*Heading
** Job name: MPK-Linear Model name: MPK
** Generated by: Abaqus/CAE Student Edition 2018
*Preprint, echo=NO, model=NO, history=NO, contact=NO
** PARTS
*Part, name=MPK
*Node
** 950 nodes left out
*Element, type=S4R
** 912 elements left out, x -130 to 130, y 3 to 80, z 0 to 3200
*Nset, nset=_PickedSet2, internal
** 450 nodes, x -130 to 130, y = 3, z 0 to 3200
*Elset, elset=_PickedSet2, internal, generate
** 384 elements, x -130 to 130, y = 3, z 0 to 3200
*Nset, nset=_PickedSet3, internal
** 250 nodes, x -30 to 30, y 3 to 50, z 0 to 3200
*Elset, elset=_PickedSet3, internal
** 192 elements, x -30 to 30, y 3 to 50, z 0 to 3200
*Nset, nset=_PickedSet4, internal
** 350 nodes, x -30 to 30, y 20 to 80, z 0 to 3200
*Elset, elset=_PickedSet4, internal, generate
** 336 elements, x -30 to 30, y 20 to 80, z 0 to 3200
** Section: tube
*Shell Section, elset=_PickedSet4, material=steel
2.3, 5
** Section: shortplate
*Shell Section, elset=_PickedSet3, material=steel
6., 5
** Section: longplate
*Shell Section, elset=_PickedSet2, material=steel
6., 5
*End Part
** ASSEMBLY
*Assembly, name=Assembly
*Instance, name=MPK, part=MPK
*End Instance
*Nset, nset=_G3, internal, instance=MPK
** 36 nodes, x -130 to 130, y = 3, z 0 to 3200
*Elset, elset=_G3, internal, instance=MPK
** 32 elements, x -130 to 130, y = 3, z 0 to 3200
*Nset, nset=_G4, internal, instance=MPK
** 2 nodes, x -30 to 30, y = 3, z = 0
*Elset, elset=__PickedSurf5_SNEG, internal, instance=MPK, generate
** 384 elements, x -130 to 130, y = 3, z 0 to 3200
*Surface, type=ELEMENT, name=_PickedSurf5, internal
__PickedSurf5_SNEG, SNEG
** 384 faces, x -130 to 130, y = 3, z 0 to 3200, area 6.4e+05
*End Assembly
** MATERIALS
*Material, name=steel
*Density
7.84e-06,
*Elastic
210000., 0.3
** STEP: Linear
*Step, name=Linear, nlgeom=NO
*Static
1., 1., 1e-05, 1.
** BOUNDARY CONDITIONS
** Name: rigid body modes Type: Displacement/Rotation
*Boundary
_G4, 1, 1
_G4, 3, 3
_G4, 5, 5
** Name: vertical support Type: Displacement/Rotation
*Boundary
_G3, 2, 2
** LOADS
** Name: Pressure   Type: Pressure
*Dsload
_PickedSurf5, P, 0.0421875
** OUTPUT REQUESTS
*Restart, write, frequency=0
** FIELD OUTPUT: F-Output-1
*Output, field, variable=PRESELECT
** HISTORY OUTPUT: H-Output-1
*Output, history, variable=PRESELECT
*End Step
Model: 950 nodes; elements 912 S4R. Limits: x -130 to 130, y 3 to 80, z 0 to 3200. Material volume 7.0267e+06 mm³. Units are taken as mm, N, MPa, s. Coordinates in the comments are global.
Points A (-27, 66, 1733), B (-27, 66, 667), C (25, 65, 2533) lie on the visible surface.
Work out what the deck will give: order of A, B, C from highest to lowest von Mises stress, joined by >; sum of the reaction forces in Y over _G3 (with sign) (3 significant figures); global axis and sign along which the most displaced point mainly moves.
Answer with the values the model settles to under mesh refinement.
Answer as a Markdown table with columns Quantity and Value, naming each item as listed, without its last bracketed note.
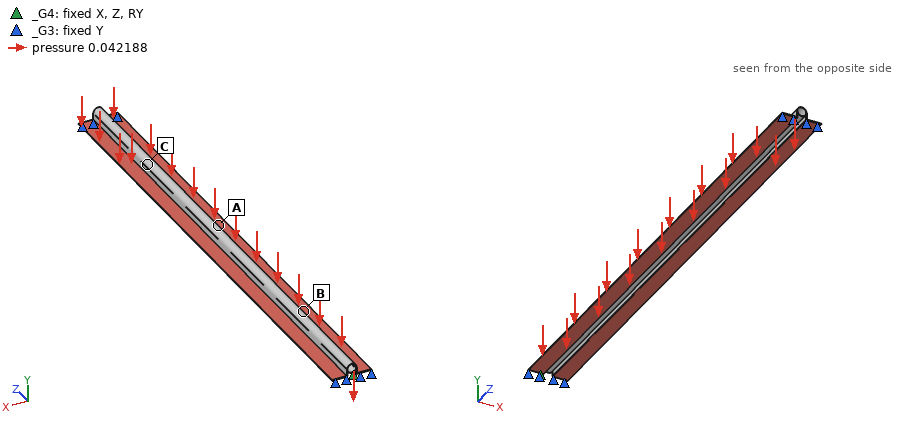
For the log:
| Quantity | Value |
|---|---|
| order of A, B, C from highest to lowest von Mises stress, joined by > | A > B > C |
| sum of the reaction forces in Y over _G3 (with sign) | 27000 N |
| global axis and sign along which the most displaced point mainly moves | -Y |
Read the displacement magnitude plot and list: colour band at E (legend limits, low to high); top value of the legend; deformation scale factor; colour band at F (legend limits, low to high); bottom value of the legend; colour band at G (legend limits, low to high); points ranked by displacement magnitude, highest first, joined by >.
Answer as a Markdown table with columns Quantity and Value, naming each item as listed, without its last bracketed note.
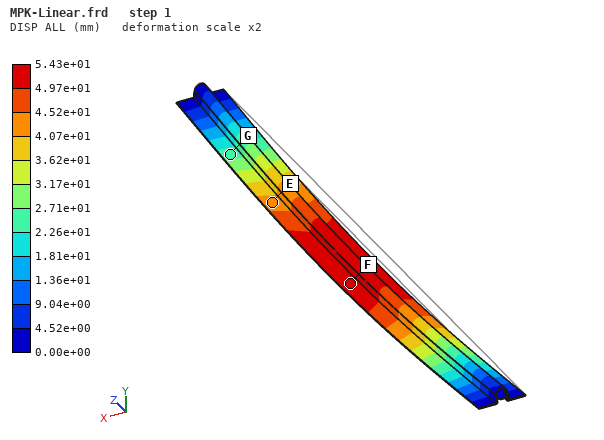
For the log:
| Quantity | Value |
|---|---|
| colour band at E | 4.07e+01 to 4.52e+01 mm |
| top value of the legend | 5.43e+01 mm |
| deformation scale factor | 2 |
| colour band at F | 4.97e+01 to 5.43e+01 mm |
| bottom value of the legend | 0.00e+00 mm |
| colour band at G | 2.26e+01 to 2.71e+01 mm |
| points ranked by displacement magnitude, highest first, joined by > | F > E > G |
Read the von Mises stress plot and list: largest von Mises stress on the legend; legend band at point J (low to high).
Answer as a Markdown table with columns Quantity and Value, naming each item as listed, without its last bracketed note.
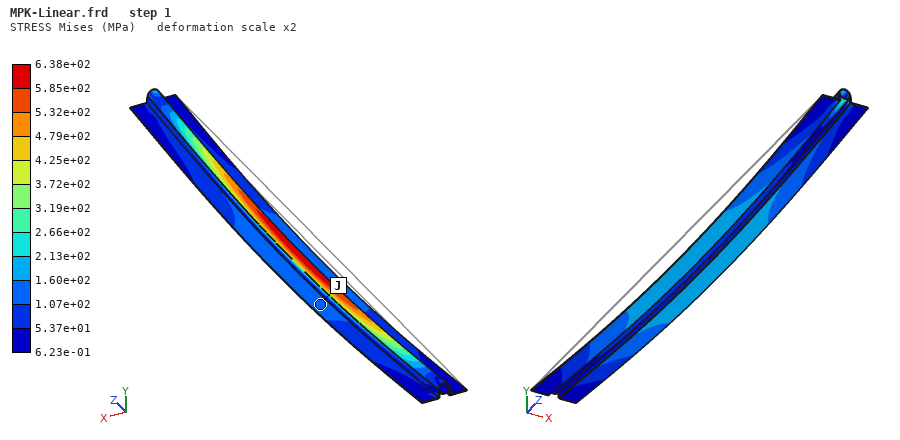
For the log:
| Quantity | Value |
|---|---|
| largest von Mises stress on the legend | 6.38e+02 MPa |
| legend band at point J | 1.07e+02 to 1.60e+02 MPa |
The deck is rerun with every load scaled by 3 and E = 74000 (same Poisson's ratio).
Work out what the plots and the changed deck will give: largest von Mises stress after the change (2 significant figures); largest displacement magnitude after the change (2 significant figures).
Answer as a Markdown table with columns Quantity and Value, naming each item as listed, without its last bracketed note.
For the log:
| Quantity | Value |
|---|---|
| largest von Mises stress after the change | 1900 MPa |
| largest displacement magnitude after the change | 460 mm |
